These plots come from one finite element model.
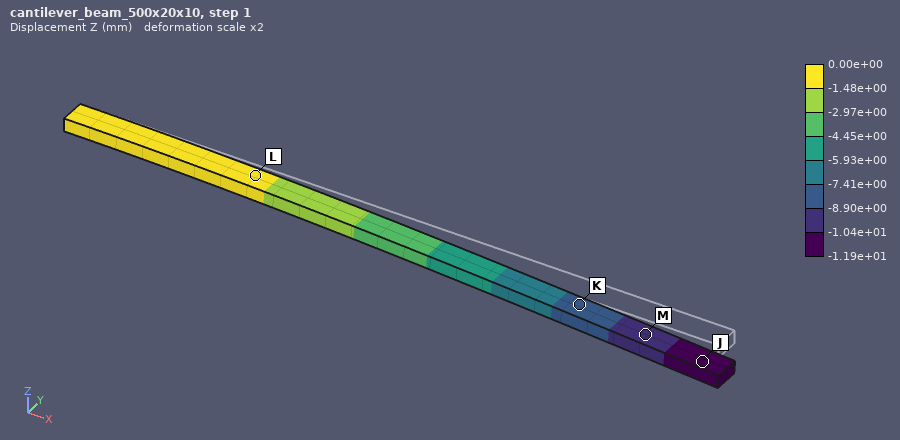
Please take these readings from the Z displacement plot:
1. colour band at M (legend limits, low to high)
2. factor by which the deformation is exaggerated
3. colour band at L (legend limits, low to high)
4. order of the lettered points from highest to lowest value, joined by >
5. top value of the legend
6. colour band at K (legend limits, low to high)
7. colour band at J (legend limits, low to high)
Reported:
-1.04e+01 to -8.90e+00 mm
2
-1.48e+00 to 0.00e+00 mm
L > K > M > J
0.00e+00 mm
-8.90e+00 to -7.41e+00 mm
-1.19e+01 to -1.04e+01 mm
